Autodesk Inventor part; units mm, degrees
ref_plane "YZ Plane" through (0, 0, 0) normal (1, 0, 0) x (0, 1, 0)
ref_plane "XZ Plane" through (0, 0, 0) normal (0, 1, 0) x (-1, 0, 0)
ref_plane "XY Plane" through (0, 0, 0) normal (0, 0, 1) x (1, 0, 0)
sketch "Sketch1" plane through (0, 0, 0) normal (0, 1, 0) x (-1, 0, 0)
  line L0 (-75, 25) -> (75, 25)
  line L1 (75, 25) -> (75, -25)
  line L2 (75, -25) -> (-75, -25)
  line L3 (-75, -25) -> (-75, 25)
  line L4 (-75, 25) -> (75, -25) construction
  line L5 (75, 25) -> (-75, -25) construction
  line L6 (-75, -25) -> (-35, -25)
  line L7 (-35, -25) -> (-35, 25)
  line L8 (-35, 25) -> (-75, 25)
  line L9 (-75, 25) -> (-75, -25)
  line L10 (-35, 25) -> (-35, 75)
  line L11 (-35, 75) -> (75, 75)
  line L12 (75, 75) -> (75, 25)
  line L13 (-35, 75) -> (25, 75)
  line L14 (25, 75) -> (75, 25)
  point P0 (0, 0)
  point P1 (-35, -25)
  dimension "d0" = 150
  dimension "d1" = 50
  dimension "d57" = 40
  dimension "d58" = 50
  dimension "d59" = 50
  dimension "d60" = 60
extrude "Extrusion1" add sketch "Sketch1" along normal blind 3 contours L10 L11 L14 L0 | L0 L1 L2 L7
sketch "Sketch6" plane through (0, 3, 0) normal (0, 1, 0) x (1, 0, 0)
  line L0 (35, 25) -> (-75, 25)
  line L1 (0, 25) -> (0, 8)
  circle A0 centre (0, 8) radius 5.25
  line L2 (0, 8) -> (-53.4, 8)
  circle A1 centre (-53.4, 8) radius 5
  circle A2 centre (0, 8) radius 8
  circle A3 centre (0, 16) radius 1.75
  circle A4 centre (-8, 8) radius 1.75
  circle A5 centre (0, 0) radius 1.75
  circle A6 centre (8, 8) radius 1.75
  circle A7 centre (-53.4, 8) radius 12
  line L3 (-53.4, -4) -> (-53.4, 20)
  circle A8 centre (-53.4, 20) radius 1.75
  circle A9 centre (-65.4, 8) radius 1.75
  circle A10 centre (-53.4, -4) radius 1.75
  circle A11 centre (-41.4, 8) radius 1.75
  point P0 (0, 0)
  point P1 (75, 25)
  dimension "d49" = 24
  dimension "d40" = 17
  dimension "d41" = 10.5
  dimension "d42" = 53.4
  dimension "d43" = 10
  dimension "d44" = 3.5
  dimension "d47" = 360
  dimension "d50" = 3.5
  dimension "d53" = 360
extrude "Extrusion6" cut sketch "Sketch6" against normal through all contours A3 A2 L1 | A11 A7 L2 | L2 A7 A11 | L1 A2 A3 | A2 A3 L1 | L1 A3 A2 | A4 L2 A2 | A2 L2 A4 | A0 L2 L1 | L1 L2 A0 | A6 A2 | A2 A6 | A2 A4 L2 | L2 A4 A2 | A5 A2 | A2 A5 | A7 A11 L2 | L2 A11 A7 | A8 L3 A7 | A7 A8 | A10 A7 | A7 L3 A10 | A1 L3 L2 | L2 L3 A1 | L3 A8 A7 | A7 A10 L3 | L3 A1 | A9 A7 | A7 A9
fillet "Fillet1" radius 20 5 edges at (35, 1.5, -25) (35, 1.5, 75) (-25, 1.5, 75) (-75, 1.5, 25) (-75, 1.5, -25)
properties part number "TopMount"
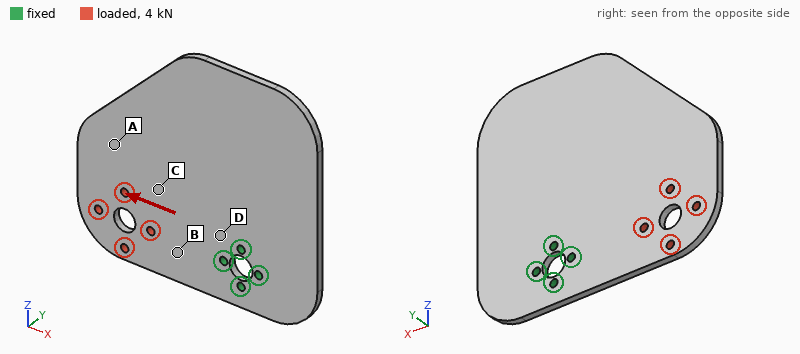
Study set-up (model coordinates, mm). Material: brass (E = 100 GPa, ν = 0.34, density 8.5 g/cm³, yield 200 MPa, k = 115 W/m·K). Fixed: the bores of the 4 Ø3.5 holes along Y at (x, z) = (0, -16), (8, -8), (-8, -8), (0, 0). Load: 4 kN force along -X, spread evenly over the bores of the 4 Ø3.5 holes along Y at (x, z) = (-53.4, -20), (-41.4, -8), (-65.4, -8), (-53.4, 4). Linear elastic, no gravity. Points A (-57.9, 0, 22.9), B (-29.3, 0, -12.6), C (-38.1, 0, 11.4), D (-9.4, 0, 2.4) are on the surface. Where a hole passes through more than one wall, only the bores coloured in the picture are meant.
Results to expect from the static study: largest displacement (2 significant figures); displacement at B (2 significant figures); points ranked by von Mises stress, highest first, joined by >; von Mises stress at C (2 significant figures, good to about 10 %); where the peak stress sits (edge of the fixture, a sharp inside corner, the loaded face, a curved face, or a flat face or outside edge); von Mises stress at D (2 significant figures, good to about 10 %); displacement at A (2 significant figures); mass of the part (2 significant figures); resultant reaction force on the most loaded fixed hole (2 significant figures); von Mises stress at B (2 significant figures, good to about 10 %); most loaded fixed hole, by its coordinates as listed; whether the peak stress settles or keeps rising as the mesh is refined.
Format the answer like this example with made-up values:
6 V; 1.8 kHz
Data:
25 µm; 10 µm; B > D > C > A; 18 MPa; edge of the fixture; 26 MPa; 9.2 µm; 240 g; 1.6 kN; 40 MPa; (-8, -8); keeps rising
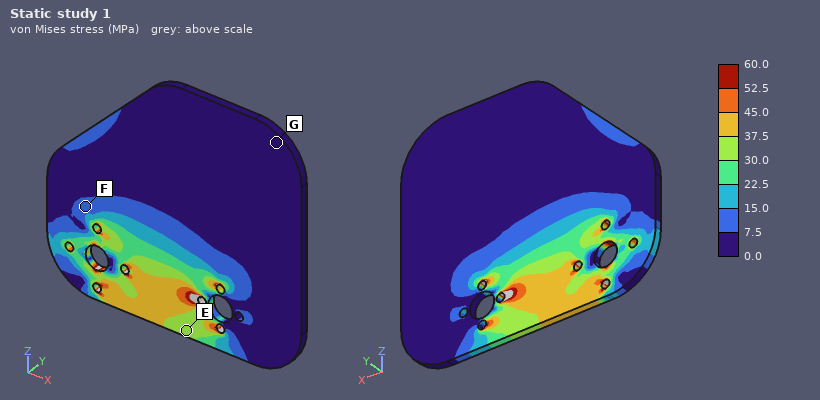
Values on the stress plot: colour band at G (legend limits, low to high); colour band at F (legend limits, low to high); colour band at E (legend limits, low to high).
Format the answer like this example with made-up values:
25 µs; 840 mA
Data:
0.0 to 7.5 MPa; 7.5 to 15.0 MPa; 30.0 to 37.5 MPa
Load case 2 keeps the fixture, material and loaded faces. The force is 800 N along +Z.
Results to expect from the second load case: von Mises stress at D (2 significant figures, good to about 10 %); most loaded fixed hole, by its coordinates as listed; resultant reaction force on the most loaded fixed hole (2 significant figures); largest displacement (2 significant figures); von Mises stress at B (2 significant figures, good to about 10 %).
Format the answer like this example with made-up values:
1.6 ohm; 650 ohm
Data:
28 MPa; (-8, -8); 1.4 kN; 44 µm; 11 MPa
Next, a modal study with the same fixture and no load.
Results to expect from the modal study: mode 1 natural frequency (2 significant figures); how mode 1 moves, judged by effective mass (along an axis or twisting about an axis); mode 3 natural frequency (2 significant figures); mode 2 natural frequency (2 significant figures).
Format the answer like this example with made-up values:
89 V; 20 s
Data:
280 Hz; along Y; 720 Hz; 350 Hz
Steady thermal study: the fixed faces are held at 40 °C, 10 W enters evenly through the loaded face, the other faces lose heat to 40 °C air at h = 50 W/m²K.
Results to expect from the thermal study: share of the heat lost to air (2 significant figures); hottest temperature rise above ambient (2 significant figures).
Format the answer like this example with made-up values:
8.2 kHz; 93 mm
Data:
53 %; 20 K
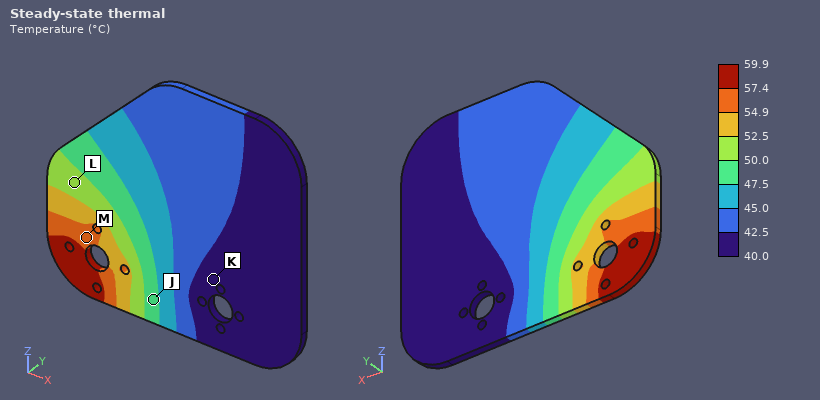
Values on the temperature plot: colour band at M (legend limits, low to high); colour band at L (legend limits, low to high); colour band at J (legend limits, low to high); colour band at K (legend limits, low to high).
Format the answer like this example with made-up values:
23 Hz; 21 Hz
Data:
54.9 to 57.4 °C; 50.0 to 52.5 °C; 47.5 to 50.0 °C; 40.0 to 42.5 °C
